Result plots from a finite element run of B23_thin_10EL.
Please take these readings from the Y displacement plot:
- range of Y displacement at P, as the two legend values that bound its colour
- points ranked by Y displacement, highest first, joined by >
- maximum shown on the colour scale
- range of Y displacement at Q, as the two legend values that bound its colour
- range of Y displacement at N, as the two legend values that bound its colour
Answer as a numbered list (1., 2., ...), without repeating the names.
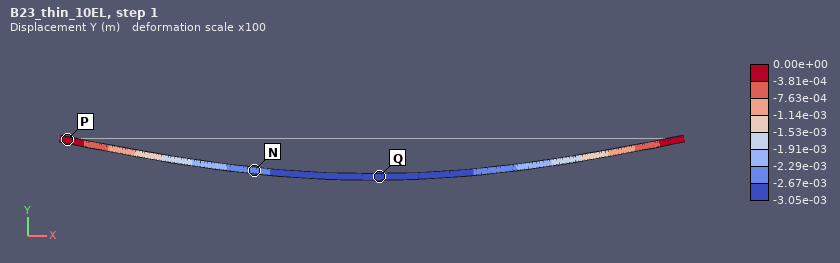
1. -3.81e-04 to 0.00e+00 m
2. P > N > Q
3. 0.00e+00 m
4. -3.05e-03 to -2.67e-03 m
5. -2.67e-03 to -2.29e-03 m
